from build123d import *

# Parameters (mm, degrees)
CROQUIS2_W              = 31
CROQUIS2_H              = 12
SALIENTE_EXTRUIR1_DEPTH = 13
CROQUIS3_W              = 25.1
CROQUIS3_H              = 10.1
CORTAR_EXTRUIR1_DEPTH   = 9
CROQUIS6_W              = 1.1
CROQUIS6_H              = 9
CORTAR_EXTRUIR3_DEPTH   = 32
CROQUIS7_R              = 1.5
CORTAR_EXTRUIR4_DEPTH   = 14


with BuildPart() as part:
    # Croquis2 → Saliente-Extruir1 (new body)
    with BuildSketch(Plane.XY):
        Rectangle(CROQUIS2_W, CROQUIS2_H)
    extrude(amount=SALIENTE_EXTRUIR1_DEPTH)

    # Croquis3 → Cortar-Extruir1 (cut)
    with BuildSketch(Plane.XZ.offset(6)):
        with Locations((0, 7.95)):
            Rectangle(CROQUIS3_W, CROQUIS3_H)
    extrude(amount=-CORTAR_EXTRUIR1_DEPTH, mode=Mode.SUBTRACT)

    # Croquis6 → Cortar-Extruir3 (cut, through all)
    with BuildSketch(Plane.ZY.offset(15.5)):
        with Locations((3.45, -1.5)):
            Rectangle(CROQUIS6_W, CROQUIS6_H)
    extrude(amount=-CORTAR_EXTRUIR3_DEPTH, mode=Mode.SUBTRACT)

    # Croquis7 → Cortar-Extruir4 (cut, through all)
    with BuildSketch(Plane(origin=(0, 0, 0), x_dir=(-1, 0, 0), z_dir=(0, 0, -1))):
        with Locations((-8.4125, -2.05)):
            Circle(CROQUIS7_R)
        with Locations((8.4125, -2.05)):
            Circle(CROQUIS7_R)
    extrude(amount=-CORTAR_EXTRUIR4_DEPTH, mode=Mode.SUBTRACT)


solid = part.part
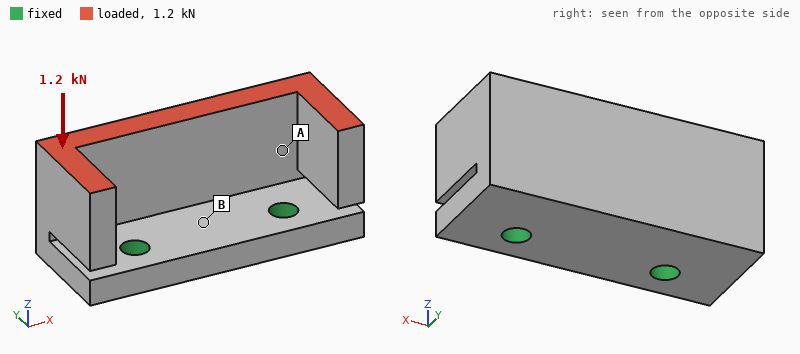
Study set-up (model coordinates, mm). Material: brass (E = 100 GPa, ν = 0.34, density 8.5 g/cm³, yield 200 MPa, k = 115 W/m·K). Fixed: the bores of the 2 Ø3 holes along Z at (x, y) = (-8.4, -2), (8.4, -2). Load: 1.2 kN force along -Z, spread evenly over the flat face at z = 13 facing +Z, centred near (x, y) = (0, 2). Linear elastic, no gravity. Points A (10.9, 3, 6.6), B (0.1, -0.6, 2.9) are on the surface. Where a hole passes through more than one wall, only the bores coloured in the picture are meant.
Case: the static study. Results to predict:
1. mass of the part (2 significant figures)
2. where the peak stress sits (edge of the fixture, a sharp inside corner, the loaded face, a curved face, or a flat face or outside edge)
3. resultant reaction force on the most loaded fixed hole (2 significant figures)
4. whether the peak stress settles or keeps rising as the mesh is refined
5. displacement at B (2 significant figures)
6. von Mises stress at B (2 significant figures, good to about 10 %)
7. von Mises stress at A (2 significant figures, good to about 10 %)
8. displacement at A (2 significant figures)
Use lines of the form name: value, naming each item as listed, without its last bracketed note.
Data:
mass of the part: 21 g
where the peak stress sits: edge of the fixture
resultant reaction force on the most loaded fixed hole: 600 N
whether the peak stress settles or keeps rising as the mesh is refined: keeps rising
displacement at B: 4.0 µm
von Mises stress at B: 20 MPa
von Mises stress at A: 58 MPa
displacement at A: 14 µm
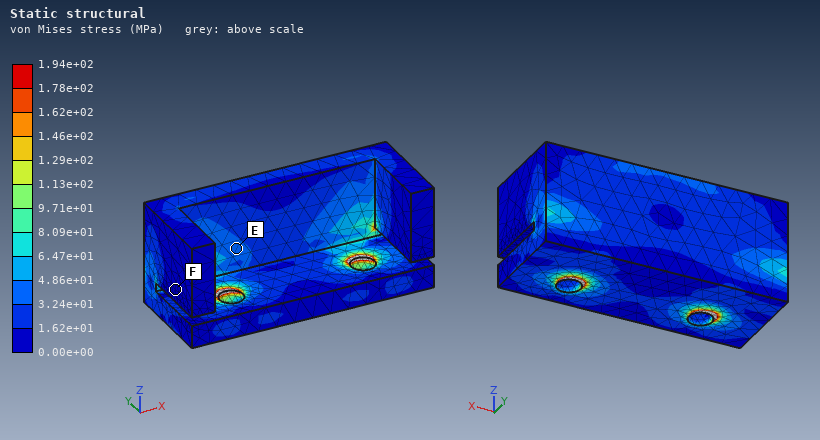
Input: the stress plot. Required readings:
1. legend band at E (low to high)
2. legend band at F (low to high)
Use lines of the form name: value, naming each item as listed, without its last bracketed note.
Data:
legend band at E: 3.24e+01 to 4.86e+01 MPa
legend band at F: 0.00e+00 to 1.62e+01 MPa
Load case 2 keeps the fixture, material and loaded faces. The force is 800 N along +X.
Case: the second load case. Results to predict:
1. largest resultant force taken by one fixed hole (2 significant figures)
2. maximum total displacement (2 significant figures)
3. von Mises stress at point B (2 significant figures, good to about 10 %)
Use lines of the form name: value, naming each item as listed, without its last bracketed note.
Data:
largest resultant force taken by one fixed hole: 640 N
maximum total displacement: 70 µm
von Mises stress at point B: 34 MPa
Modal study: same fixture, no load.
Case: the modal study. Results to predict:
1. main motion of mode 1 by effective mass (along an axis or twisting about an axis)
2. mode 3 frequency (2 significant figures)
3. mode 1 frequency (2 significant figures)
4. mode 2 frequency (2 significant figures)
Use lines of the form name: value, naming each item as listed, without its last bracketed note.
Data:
main motion of mode 1 by effective mass: along Y
mode 3 frequency: 9100 Hz
mode 1 frequency: 4900 Hz
mode 2 frequency: 6200 Hz
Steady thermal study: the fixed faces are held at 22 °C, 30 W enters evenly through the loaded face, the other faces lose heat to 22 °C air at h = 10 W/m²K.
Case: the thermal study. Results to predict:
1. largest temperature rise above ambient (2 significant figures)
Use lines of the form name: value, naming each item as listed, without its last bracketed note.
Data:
largest temperature rise above ambient: 54 K
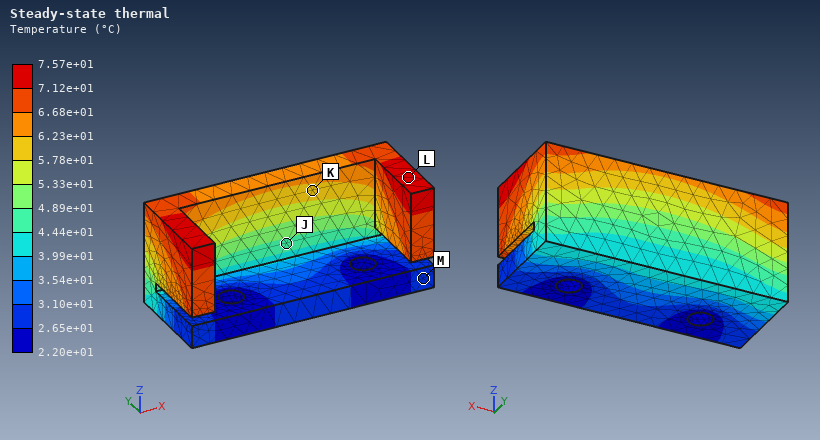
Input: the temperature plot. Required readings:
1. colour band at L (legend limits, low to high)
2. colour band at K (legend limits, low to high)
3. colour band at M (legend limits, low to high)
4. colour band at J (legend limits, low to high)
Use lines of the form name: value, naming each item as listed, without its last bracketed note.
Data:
colour band at L: 7.12e+01 to 7.57e+01 °C
colour band at K: 5.78e+01 to 6.23e+01 °C
colour band at M: 2.65e+01 to 3.10e+01 °C
colour band at J: 4.44e+01 to 4.89e+01 °C
